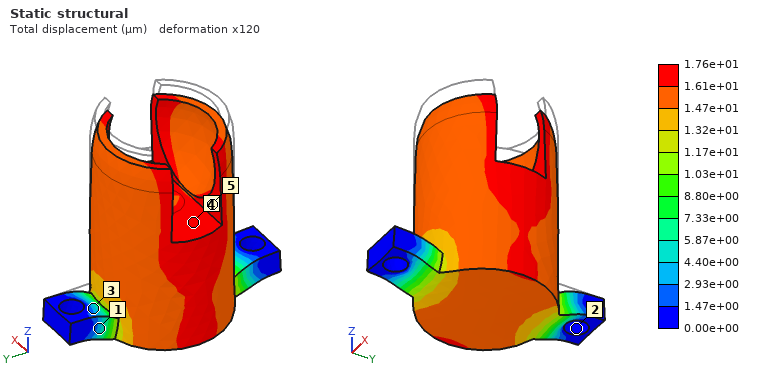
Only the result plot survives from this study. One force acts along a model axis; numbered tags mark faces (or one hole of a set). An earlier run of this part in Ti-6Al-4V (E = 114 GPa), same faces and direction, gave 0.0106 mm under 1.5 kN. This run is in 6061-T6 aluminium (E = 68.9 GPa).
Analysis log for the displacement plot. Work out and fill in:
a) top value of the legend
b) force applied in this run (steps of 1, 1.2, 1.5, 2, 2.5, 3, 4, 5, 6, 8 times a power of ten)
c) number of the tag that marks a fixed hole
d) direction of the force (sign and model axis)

1.76e+01 µm
1.5 kN
2
-Z
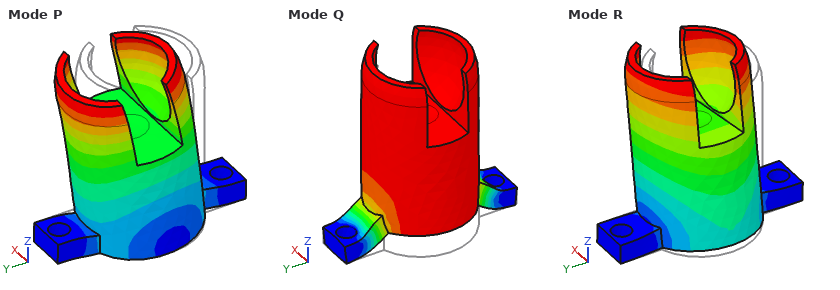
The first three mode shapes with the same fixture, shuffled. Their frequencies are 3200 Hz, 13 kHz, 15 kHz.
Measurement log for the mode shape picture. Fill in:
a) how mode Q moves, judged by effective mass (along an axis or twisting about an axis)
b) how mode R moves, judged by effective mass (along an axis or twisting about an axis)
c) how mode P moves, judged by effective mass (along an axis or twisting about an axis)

along Z
along X
along Y
